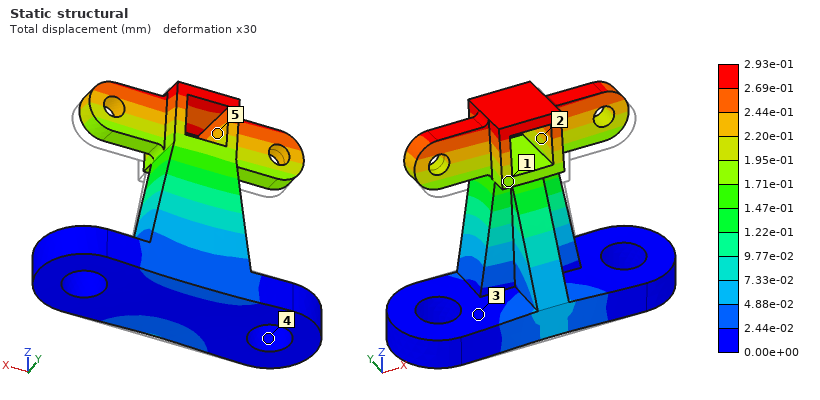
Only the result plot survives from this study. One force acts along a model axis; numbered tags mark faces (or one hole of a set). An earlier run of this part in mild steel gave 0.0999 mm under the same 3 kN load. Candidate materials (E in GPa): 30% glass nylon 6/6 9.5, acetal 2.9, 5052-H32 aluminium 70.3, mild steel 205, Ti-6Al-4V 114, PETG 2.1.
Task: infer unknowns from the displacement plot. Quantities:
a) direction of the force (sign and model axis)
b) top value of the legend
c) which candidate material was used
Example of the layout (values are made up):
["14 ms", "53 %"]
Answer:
["+Y", "2.93e-01 mm", "5052-H32 aluminium"]
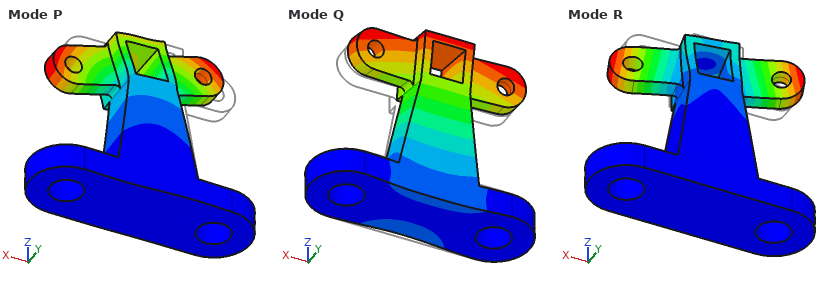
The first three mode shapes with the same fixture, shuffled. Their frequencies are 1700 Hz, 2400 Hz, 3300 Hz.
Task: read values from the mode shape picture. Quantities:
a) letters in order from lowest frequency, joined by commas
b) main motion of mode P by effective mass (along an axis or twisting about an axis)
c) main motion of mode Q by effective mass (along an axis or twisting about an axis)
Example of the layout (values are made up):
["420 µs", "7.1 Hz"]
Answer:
["Q, P, R", "along X", "along Y"]
